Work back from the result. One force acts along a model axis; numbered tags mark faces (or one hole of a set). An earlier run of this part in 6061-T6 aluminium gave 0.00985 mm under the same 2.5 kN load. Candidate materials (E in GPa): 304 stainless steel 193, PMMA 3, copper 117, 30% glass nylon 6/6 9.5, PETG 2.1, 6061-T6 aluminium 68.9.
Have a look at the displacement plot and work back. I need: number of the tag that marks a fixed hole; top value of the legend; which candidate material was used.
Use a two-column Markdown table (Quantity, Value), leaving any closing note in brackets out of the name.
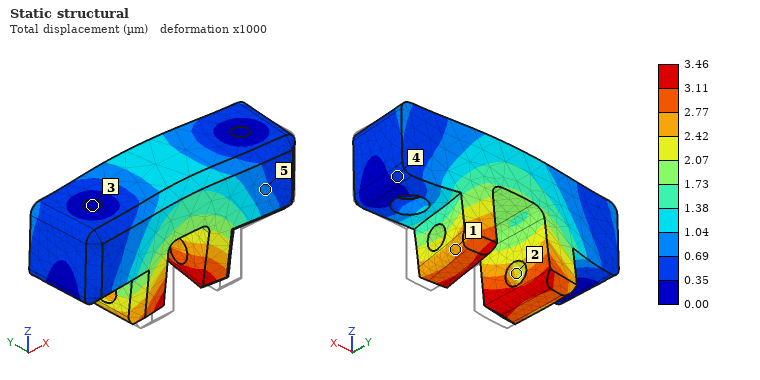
| Quantity | Value |
|---|---|
| number of the tag that marks a fixed hole | 3 |
| top value of the legend | 3.46 µm |
| which candidate material was used | 304 stainless steel |
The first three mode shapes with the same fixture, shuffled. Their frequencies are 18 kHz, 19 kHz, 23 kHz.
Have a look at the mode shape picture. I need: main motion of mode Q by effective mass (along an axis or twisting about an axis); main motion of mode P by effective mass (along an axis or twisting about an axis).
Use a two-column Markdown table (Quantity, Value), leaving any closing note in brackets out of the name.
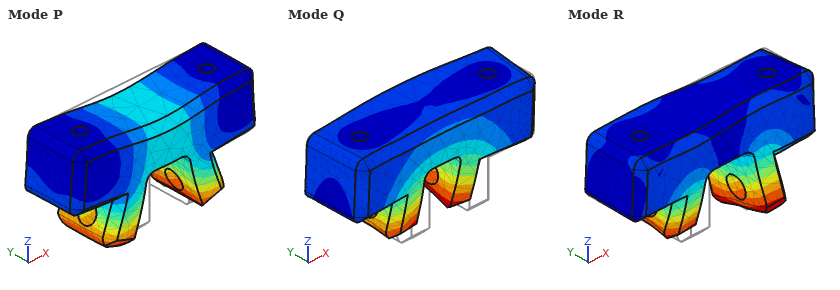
| Quantity | Value |
|---|---|
| main motion of mode Q by effective mass | along Y |
| main motion of mode P by effective mass | along Z |
